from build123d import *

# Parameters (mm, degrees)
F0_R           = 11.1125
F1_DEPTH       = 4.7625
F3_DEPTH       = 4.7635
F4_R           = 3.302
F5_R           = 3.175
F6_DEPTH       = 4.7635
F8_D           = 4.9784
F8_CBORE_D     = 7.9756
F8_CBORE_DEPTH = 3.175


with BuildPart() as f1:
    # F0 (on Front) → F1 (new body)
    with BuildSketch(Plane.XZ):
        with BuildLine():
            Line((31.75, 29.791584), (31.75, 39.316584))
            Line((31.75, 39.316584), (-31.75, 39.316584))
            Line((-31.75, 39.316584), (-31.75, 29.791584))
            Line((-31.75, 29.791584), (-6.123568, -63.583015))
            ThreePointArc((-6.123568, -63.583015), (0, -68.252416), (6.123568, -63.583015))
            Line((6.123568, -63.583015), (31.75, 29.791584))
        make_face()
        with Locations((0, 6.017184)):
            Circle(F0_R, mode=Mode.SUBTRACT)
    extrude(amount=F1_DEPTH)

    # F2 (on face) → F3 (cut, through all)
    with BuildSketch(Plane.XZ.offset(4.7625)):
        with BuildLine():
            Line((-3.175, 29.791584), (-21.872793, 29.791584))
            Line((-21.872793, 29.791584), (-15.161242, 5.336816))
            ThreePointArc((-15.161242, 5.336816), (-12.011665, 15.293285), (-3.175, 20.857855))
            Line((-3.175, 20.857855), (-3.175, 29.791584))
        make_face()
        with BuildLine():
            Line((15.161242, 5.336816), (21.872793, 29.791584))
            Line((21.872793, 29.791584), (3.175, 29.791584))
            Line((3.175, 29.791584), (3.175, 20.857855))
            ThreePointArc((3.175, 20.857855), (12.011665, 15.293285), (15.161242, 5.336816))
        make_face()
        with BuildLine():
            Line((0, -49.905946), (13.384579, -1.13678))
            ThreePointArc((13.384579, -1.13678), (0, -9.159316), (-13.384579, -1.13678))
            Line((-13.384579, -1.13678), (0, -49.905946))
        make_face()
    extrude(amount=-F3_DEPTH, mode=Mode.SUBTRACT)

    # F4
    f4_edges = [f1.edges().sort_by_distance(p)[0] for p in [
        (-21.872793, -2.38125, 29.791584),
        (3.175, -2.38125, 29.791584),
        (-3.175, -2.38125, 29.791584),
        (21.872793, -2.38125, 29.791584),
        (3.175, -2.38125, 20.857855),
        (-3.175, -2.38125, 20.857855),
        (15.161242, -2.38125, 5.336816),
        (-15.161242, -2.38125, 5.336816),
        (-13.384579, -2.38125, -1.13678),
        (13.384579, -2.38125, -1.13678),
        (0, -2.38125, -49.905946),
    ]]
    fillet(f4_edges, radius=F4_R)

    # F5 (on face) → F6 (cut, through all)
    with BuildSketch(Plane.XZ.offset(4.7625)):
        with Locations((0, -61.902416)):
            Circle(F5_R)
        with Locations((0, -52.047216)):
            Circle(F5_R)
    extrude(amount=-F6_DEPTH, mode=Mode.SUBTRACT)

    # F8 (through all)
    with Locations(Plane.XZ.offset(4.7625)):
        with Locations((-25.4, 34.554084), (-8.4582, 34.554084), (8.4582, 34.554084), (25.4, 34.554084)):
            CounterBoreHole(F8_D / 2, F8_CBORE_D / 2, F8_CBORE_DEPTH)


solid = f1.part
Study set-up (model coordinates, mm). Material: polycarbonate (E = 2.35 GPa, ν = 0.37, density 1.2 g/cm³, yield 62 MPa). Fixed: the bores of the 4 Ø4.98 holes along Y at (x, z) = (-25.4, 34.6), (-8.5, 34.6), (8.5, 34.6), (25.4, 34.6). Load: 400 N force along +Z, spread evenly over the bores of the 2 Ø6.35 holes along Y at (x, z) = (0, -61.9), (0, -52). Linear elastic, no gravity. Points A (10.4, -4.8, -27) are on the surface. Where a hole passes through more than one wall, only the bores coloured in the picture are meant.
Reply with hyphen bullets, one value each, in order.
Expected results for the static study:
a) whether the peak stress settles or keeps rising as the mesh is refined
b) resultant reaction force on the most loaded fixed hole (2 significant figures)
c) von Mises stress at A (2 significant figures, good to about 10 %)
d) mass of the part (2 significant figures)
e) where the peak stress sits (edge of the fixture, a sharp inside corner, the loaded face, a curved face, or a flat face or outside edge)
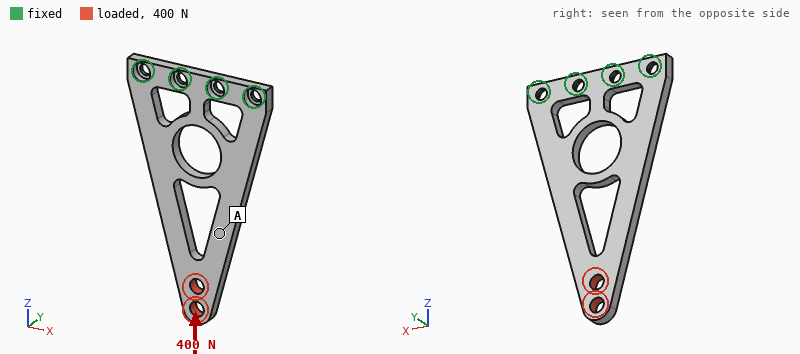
- keeps rising
- 170 N
- 4.6 MPa
- 15 g
- edge of the fixture
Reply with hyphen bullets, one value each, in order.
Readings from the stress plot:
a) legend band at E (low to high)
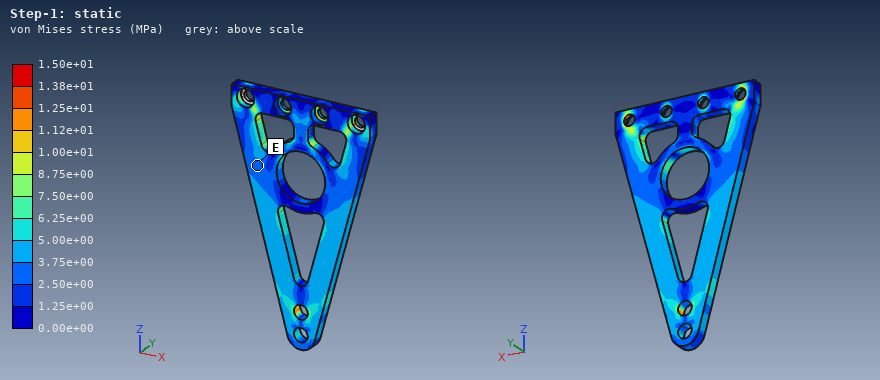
- 2.50e+00 to 3.75e+00 MPa
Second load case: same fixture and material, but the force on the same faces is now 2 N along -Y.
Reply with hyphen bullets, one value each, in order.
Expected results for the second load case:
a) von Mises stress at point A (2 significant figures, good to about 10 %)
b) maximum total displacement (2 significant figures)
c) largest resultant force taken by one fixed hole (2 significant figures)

- 0.84 MPa
- 1.3 mm
- 2.7 N
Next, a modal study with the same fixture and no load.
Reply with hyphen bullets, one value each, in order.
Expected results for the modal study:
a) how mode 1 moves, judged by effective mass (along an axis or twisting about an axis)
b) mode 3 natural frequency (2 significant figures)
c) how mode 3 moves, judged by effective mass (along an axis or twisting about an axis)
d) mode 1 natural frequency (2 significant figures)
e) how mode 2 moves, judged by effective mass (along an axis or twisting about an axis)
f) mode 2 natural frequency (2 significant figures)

- along Y
- 660 Hz
- twisting about Z
- 120 Hz
- along Y
- 630 Hz
